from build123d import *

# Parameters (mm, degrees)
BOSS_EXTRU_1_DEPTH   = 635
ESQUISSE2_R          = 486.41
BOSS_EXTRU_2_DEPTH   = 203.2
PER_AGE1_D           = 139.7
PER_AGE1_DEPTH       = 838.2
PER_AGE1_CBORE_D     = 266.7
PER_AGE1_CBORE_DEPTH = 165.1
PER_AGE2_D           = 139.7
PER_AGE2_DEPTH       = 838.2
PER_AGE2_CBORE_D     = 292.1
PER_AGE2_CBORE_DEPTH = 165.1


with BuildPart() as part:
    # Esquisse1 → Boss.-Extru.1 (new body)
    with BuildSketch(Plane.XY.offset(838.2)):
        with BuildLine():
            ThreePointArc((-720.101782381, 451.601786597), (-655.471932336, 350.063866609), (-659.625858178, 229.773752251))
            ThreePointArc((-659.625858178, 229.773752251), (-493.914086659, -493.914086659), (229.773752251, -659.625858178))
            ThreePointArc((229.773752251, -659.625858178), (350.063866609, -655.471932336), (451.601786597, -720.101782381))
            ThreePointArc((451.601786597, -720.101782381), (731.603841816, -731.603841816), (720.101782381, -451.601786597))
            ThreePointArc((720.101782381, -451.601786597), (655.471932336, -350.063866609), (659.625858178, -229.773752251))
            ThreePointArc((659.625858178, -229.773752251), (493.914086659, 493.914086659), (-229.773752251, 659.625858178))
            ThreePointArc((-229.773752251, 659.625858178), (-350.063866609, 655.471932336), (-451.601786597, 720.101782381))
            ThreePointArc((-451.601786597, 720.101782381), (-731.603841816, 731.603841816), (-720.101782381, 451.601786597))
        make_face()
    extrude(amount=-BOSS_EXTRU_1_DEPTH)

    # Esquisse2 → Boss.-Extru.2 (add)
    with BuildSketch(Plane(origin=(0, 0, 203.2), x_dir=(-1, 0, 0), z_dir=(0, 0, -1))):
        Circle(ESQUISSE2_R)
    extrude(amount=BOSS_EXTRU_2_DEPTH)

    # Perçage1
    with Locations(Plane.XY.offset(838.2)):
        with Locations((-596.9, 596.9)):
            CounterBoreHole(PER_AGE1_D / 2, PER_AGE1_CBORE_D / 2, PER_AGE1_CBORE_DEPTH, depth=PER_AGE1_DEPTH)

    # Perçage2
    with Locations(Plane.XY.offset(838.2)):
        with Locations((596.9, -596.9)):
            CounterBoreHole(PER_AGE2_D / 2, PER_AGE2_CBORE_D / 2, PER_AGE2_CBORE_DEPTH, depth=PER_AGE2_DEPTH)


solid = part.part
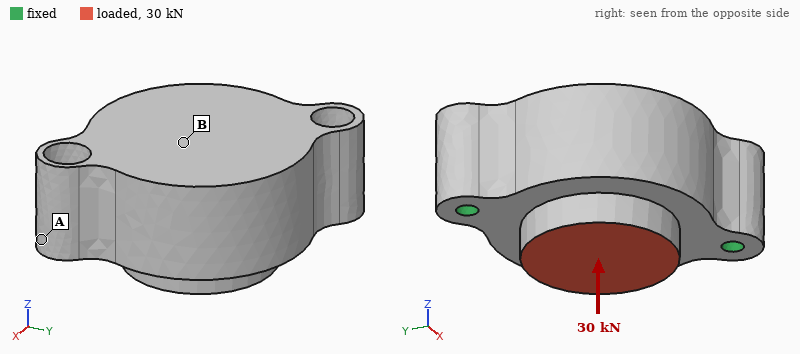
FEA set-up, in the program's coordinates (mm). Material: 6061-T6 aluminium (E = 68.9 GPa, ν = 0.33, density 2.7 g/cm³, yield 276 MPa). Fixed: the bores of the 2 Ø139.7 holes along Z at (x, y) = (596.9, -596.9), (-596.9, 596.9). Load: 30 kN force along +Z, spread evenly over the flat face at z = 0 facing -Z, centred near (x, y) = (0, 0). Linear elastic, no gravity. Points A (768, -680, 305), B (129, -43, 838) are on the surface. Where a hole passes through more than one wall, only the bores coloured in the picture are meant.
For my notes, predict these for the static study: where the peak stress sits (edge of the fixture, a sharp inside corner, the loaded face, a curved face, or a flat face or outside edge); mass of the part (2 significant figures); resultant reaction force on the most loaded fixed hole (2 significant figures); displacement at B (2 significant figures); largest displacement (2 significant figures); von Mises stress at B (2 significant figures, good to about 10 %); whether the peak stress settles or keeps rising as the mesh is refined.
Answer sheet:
edge of the fixture
3400 kg
15 kN
1.5 µm
1.9 µm
0.075 MPa
keeps rising
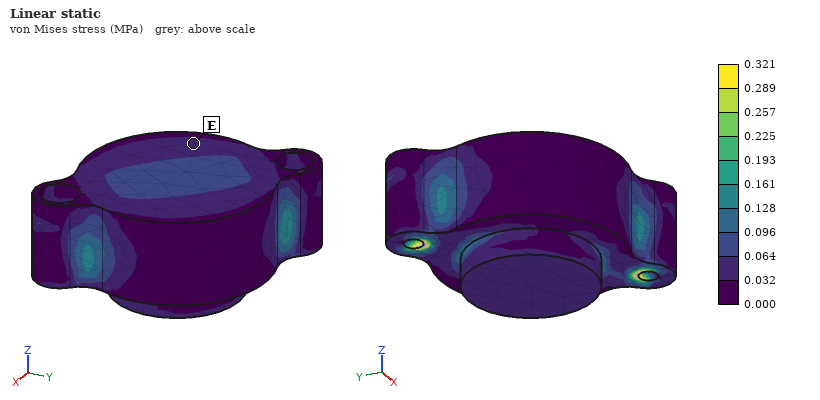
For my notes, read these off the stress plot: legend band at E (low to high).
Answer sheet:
0.032 to 0.064 MPa
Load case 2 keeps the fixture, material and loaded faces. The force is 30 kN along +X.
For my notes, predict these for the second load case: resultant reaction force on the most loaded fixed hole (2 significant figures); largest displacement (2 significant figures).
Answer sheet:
16 kN
6.3 µm
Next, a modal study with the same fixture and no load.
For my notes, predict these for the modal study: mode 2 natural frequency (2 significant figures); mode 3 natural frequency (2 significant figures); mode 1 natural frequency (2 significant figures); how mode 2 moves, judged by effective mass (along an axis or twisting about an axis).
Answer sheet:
410 Hz
470 Hz
260 Hz
along Z
